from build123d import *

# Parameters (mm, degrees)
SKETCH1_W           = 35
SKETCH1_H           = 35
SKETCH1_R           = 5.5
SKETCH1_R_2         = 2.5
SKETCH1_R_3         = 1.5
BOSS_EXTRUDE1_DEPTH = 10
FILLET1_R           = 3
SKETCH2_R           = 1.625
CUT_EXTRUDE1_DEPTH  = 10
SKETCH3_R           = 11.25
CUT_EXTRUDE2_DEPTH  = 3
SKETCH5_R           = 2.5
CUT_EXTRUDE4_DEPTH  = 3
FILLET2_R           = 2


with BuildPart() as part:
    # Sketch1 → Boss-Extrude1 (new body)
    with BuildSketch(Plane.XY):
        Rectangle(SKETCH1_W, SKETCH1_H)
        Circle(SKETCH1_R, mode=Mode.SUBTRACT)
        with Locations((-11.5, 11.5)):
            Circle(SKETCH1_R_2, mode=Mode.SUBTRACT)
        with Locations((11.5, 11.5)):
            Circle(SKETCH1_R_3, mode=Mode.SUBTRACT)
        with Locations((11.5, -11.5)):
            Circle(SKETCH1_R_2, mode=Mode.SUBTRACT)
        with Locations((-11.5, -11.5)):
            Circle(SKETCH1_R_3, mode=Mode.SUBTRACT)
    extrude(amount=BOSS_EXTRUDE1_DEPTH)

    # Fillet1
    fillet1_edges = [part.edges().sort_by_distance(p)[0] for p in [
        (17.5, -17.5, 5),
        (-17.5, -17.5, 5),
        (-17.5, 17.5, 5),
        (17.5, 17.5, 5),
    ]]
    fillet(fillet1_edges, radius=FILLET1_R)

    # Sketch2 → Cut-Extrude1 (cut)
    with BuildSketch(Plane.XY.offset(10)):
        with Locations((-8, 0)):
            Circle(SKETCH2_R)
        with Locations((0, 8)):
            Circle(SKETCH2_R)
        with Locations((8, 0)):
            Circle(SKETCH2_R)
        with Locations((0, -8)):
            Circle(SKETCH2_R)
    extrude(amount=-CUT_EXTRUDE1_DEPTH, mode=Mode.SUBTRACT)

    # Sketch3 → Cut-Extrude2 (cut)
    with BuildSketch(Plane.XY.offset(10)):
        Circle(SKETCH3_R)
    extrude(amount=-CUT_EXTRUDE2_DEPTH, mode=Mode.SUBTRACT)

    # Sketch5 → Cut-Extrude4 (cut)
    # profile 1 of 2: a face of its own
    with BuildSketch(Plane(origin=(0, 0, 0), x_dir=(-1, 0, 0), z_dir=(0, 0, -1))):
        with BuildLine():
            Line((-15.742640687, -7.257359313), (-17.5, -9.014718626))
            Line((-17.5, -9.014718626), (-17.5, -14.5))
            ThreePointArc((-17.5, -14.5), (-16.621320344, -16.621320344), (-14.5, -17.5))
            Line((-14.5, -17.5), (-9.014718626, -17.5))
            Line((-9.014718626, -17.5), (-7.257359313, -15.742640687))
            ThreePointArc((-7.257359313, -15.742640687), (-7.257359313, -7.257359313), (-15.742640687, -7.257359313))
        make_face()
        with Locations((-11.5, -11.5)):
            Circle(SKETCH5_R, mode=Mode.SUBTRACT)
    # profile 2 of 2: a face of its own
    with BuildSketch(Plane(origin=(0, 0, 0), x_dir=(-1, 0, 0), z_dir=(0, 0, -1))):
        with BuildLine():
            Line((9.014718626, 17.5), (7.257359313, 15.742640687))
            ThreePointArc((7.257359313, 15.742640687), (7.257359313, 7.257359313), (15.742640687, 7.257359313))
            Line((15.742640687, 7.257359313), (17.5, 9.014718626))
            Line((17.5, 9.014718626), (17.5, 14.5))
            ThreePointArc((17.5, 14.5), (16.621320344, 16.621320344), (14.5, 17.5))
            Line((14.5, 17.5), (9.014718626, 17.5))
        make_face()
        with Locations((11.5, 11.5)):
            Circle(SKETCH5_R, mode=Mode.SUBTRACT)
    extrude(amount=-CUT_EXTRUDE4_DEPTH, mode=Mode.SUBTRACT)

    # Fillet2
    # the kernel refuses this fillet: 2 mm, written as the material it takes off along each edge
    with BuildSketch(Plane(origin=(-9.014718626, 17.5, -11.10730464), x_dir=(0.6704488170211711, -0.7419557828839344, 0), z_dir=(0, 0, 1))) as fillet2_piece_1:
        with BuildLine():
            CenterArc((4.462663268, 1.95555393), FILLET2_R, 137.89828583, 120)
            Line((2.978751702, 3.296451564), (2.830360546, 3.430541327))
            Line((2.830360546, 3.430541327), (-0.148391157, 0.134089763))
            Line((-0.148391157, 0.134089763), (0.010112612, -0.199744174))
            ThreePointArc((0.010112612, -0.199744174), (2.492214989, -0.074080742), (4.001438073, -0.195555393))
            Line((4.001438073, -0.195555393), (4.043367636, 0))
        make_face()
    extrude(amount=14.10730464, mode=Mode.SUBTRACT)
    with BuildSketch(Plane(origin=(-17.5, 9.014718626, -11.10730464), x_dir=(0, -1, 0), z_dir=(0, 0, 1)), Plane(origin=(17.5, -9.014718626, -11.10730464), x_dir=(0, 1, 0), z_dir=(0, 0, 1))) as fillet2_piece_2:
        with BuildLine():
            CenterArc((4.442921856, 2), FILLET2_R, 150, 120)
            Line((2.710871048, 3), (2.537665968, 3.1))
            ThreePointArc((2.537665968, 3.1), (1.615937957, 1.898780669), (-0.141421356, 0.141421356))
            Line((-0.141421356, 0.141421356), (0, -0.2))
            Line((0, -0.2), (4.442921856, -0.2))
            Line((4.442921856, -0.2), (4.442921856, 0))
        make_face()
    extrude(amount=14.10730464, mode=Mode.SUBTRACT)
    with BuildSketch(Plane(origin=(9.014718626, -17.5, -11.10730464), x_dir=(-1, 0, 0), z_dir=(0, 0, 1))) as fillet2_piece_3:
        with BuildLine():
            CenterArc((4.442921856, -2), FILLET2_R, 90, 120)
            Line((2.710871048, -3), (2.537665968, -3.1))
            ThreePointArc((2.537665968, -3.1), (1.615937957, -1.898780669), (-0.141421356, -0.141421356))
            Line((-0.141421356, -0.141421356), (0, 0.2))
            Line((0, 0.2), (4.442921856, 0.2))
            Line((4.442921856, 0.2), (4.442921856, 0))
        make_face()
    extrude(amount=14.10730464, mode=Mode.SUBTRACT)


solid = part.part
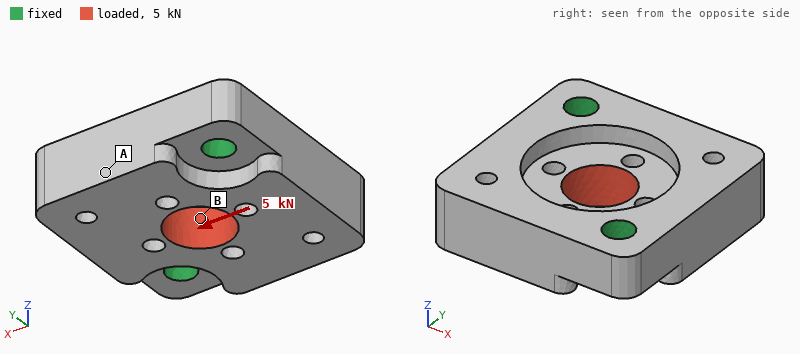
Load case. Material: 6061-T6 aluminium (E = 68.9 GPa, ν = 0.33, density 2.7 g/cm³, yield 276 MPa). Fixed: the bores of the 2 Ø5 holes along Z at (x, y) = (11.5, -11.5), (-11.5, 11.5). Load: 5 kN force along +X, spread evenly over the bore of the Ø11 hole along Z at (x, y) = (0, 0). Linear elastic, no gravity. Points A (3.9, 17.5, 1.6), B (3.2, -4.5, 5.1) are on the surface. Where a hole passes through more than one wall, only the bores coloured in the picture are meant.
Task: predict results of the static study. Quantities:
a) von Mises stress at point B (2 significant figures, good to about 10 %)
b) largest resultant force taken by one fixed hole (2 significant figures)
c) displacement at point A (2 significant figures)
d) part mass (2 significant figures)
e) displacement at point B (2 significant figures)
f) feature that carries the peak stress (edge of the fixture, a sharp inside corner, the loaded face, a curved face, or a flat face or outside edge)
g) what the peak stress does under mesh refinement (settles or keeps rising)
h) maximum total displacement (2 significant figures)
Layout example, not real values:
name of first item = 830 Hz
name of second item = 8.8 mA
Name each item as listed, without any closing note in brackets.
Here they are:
von Mises stress at point B = 36 MPa
largest resultant force taken by one fixed hole = 2.5 kN
displacement at point A = 12 µm
part mass = 24 g
displacement at point B = 8.3 µm
feature that carries the peak stress = edge of the fixture
what the peak stress does under mesh refinement = keeps rising
maximum total displacement = 21 µm
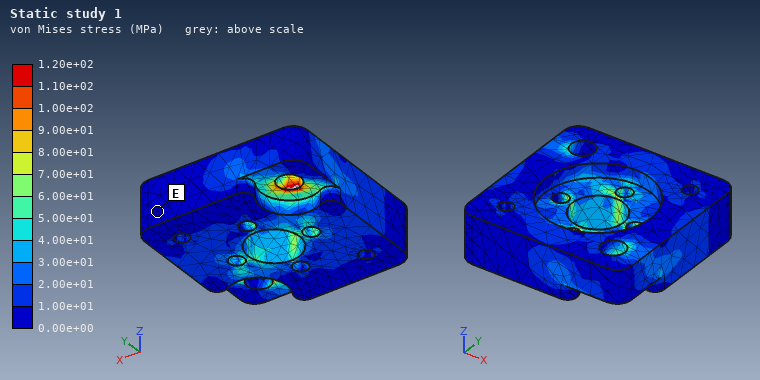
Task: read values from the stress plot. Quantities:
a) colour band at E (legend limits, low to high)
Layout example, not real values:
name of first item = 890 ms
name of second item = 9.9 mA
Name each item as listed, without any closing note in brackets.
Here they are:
colour band at E = 0.00e+00 to 1.00e+01 MPa
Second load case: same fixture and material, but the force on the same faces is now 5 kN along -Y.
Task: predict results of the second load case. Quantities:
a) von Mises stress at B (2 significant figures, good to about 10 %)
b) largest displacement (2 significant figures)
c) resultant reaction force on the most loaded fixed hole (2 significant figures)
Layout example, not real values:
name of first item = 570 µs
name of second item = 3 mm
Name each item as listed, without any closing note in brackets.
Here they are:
von Mises stress at B = 32 MPa
largest displacement = 21 µm
resultant reaction force on the most loaded fixed hole = 2.5 kN
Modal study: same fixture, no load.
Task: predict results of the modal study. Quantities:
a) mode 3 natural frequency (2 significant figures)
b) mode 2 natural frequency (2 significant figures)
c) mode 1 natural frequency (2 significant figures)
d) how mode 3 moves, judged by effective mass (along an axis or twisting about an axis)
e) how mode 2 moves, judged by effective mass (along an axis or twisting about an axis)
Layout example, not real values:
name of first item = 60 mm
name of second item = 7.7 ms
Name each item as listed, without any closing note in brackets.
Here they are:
mode 3 natural frequency = 32 kHz
mode 2 natural frequency = 13 kHz
mode 1 natural frequency = 10 kHz
how mode 3 moves, judged by effective mass = twisting about Z
how mode 2 moves, judged by effective mass = along Z
